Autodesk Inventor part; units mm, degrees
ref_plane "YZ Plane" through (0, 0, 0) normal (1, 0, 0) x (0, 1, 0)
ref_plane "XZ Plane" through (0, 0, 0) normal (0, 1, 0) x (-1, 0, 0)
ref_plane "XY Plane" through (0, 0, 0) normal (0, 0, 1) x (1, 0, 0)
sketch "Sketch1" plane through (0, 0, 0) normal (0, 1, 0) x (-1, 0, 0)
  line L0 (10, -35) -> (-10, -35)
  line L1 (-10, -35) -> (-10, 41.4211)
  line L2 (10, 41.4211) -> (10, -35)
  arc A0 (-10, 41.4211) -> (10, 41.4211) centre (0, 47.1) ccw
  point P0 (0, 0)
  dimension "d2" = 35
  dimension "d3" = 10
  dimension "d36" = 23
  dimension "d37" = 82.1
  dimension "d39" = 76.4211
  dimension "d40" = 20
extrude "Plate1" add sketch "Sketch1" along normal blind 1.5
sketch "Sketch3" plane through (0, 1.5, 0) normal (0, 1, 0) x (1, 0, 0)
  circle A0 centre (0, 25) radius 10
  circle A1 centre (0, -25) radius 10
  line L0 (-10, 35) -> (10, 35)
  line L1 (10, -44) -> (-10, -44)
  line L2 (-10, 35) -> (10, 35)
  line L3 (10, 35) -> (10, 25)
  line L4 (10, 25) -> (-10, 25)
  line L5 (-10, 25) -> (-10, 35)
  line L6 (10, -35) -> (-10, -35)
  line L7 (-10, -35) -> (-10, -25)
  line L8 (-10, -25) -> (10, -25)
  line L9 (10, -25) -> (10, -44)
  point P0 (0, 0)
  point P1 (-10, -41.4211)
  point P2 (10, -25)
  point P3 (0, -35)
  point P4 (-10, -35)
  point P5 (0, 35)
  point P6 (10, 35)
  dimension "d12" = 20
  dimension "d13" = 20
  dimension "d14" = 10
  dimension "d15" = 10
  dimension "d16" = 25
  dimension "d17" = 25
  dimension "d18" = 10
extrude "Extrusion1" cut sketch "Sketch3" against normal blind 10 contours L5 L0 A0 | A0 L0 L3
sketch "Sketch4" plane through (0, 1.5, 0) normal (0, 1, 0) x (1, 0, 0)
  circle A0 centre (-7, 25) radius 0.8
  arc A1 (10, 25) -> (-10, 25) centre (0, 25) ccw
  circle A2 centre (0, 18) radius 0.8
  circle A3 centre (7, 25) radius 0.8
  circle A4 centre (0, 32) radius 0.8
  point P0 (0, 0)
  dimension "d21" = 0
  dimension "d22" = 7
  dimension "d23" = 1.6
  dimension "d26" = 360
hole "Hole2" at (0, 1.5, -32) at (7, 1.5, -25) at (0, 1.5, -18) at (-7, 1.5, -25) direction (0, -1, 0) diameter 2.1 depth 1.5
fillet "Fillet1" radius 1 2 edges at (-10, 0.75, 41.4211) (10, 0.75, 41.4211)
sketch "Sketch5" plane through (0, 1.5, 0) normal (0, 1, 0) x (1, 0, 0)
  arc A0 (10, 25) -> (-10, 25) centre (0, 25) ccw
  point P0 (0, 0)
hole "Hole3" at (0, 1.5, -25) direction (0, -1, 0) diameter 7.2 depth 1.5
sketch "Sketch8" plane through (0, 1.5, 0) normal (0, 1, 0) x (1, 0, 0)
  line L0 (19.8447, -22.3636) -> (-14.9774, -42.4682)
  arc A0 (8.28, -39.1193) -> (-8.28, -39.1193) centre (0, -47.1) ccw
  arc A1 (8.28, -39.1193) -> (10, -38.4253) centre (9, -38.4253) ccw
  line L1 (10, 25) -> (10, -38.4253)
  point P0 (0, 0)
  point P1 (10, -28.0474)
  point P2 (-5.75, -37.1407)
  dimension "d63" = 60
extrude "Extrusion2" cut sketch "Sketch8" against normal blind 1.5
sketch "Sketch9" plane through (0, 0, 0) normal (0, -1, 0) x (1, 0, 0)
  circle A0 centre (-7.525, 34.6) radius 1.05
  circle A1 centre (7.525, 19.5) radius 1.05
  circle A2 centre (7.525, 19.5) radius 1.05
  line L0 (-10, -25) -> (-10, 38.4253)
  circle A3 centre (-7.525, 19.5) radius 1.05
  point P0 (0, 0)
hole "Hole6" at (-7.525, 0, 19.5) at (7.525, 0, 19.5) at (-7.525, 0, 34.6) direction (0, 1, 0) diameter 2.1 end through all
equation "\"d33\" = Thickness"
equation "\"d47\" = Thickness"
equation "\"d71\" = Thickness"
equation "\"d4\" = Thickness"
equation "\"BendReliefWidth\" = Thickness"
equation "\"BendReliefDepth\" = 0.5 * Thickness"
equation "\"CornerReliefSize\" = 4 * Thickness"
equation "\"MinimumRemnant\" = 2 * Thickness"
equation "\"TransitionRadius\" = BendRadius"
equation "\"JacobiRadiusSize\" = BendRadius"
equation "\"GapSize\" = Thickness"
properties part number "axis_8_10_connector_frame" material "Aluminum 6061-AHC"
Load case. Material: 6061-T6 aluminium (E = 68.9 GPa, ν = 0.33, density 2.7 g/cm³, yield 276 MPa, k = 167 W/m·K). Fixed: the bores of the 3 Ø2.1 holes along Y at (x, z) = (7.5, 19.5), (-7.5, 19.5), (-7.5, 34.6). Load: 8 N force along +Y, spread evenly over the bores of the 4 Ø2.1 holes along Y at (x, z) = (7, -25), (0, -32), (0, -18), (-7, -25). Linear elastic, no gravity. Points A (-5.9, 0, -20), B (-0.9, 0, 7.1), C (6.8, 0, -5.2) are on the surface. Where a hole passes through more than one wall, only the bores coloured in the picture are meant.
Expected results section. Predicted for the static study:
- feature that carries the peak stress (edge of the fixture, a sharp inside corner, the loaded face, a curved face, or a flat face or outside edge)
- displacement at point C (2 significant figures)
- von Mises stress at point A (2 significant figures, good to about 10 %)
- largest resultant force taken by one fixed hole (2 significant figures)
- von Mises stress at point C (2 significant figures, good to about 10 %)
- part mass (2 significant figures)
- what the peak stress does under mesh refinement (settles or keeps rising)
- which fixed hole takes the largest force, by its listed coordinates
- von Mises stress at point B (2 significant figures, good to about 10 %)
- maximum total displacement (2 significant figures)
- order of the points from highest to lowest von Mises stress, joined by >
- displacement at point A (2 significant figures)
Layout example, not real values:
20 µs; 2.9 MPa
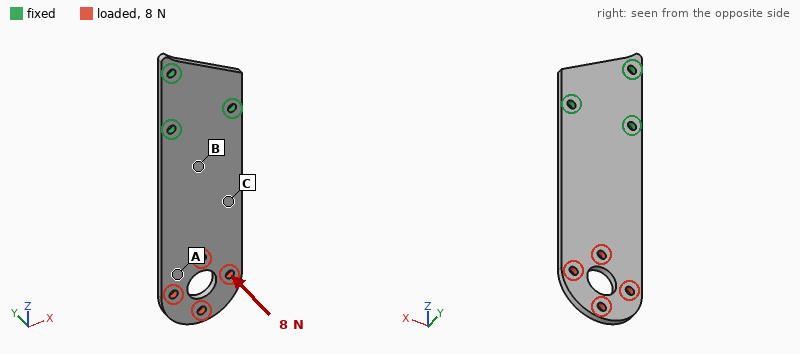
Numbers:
edge of the fixture; 0.23 mm; 7.5 MPa; 6.9 N; 21 MPa; 5.1 g; keeps rising; (-7.5, 19.5); 33 MPa; 0.81 mm; B > C > A; 0.50 mm
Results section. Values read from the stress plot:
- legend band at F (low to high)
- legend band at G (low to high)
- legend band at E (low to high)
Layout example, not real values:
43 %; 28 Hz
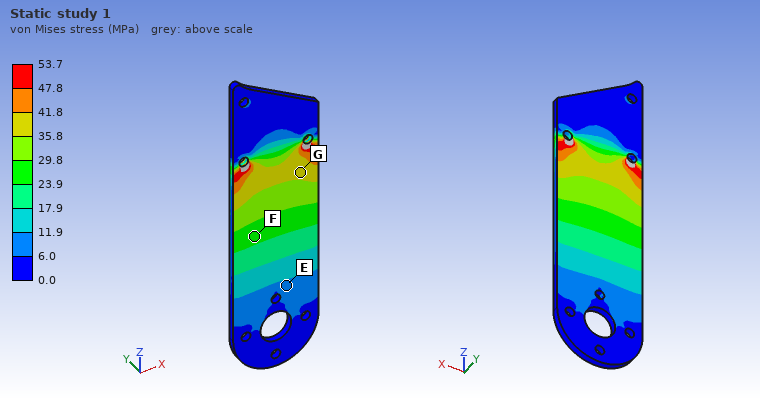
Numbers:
23.9 to 29.8 MPa; 35.8 to 41.8 MPa; 6.0 to 11.9 MPa
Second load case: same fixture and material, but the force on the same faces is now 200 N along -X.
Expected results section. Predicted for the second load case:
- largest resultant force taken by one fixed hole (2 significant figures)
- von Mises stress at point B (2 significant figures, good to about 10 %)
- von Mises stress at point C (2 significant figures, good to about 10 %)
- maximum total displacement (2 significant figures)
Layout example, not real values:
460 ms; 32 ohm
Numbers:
560 N; 18 MPa; 28 MPa; 0.13 mm
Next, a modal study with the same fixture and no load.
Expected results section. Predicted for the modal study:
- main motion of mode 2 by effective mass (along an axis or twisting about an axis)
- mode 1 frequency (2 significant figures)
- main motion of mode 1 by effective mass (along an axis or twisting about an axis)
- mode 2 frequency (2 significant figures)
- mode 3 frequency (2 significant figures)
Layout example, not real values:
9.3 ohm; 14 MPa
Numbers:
twisting about Z; 480 Hz; along Y; 2600 Hz; 2800 Hz
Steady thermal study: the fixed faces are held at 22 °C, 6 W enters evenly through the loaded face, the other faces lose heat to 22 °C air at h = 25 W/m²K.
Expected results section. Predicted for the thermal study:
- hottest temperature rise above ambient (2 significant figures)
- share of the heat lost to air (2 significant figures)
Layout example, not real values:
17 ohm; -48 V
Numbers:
50 K; 23 %
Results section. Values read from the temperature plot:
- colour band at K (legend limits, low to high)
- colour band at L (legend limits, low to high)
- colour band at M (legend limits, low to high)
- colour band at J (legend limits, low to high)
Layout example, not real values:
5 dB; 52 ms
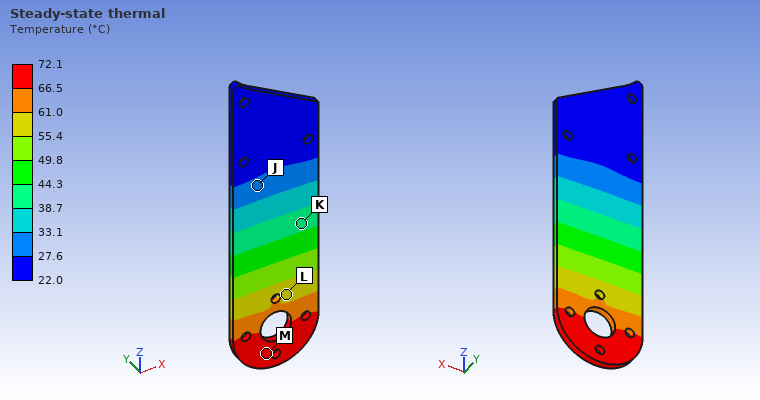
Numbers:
38.7 to 44.3 °C; 55.4 to 61.0 °C; 66.5 to 72.1 °C; 27.6 to 33.1 °C
